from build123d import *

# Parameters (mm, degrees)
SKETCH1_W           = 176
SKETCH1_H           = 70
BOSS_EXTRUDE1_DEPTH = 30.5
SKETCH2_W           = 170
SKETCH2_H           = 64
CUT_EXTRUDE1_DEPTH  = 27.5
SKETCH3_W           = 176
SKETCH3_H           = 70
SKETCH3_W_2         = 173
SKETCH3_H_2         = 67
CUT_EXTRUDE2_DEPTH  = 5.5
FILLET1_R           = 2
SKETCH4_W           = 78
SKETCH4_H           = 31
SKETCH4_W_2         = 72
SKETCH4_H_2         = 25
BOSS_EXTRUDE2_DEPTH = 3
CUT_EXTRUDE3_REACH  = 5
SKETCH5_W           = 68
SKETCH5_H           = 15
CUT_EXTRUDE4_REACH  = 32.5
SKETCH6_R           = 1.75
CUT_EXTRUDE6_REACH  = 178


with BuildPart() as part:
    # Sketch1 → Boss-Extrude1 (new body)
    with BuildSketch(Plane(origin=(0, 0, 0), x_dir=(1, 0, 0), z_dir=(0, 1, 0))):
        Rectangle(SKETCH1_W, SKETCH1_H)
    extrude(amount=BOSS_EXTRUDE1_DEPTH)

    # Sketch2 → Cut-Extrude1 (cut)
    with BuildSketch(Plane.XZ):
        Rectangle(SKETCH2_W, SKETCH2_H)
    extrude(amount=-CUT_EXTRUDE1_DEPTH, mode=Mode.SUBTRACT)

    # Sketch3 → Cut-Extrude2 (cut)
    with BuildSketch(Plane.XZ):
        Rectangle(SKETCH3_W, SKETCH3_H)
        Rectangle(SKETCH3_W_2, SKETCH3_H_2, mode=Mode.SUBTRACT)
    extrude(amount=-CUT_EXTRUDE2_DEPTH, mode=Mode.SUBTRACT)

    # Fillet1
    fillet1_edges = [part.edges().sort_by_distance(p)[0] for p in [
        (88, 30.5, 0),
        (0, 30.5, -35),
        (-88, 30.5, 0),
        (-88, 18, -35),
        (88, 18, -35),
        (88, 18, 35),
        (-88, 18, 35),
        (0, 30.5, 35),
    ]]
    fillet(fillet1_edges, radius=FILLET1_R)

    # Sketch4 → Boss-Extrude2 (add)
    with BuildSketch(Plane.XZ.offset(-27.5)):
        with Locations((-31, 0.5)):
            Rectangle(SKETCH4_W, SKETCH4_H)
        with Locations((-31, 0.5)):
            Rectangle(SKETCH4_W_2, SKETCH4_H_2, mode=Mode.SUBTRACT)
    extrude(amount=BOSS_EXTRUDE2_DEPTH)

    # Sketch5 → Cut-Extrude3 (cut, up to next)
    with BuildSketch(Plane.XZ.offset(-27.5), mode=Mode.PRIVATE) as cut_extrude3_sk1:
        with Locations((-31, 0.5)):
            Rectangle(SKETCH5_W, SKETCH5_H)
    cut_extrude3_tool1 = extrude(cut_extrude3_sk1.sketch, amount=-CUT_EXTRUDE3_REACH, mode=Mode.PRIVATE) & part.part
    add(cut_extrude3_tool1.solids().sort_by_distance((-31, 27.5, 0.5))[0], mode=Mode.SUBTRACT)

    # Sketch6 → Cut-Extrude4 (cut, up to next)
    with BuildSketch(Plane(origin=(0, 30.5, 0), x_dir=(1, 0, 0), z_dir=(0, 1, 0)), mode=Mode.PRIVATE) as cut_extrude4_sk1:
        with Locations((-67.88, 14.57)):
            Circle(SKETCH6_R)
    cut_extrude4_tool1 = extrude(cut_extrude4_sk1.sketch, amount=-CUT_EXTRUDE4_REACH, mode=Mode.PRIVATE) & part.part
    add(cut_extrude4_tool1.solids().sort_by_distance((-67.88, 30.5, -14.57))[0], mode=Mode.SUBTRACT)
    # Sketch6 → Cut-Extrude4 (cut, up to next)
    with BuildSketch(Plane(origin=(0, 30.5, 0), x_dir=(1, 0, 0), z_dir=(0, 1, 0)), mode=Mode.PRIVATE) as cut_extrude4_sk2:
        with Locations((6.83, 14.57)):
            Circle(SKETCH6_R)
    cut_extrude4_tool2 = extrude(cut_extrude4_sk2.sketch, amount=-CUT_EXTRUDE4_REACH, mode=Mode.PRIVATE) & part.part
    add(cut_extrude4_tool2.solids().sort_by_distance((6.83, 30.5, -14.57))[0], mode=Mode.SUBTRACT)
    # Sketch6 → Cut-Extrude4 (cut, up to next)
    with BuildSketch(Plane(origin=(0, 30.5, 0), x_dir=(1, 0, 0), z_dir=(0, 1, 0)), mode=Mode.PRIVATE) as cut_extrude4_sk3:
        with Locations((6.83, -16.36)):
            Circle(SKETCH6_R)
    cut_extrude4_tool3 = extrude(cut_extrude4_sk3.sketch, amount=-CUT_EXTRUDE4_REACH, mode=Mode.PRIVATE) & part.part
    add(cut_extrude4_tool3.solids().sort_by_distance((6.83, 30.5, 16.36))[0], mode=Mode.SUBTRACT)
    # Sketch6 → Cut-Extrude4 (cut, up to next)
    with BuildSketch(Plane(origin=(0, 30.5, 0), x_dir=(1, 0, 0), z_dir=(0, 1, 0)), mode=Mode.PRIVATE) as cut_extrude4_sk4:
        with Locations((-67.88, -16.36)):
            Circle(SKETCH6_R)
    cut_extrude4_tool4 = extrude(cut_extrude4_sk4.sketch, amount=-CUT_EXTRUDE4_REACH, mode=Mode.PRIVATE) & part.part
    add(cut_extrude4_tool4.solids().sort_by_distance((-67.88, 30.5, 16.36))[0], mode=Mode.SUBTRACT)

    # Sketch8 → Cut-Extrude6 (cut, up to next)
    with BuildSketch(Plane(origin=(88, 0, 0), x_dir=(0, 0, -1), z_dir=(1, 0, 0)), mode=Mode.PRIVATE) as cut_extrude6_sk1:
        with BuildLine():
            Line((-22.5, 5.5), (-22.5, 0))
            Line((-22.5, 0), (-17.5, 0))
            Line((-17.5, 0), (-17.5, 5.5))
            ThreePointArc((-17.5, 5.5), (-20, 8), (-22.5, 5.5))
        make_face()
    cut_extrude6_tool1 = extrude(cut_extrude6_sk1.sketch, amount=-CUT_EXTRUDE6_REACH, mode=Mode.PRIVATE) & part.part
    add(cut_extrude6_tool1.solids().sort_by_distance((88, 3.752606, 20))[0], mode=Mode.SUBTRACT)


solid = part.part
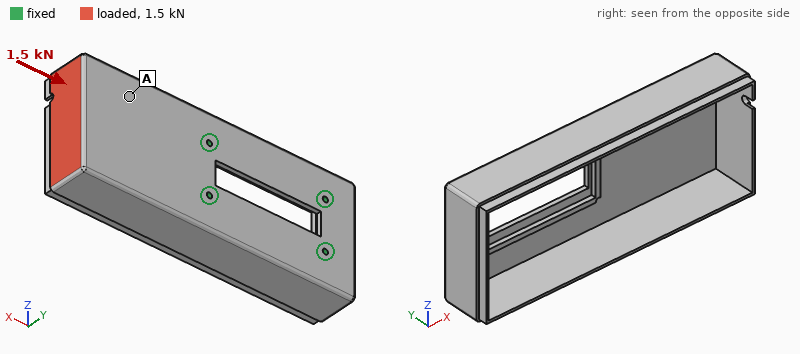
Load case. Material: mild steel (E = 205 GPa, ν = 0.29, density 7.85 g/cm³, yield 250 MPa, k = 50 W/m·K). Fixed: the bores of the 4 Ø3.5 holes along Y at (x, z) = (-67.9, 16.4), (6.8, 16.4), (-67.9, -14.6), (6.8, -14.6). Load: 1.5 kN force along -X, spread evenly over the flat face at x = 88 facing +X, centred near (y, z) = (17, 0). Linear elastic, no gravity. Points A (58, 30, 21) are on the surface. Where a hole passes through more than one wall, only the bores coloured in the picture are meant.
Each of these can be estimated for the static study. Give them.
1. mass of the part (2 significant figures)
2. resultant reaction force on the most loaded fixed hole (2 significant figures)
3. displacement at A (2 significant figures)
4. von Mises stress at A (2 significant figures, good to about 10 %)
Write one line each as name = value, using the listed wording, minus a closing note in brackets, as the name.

mass of the part = 550 g
resultant reaction force on the most loaded fixed hole = 510 N
displacement at A = 0.017 mm
von Mises stress at A = 7.2 MPa
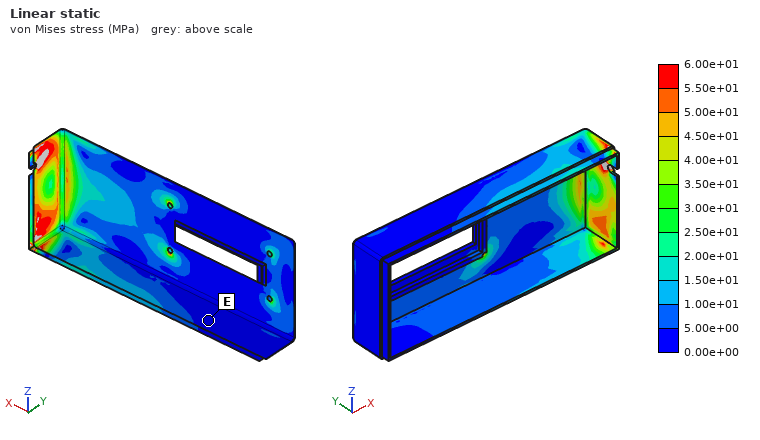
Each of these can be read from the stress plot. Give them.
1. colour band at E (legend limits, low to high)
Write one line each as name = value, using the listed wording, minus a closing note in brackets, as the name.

colour band at E = 0.00e+00 to 5.00e+00 MPa
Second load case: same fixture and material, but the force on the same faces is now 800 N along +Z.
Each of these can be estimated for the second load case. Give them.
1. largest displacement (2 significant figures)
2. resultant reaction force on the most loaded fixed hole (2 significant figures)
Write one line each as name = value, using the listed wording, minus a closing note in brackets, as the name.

largest displacement = 0.14 mm
resultant reaction force on the most loaded fixed hole = 1.5 kN
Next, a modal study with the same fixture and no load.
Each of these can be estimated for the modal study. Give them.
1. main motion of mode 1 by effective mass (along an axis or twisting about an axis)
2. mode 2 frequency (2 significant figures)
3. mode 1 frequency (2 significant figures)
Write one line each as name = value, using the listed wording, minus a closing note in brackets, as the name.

main motion of mode 1 by effective mass = along Y
mode 2 frequency = 910 Hz
mode 1 frequency = 830 Hz
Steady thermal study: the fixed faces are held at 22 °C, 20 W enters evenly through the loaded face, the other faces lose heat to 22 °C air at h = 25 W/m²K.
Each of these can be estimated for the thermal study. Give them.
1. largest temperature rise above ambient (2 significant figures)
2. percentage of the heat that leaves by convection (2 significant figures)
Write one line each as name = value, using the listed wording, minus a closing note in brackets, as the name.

largest temperature rise above ambient = 61 K
percentage of the heat that leaves by convection = 76 %
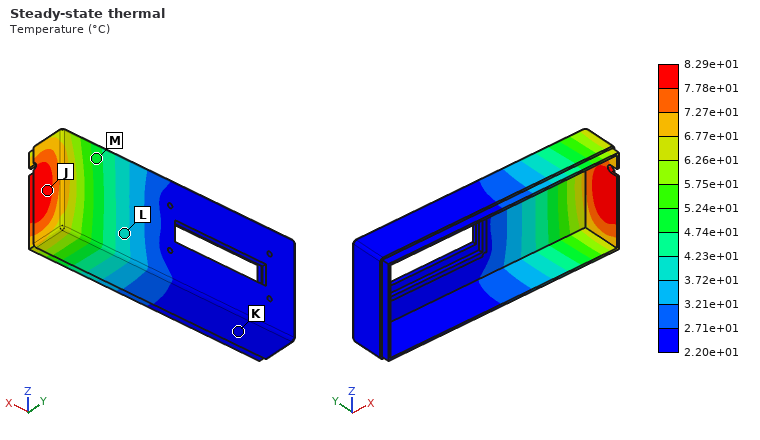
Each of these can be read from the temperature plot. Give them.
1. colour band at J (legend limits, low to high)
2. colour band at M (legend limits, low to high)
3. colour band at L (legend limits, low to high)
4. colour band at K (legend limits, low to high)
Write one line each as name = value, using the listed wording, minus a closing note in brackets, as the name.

colour band at J = 7.78e+01 to 8.29e+01 °C
colour band at M = 4.74e+01 to 5.24e+01 °C
colour band at L = 3.72e+01 to 4.23e+01 °C
colour band at K = 2.20e+01 to 2.71e+01 °C
